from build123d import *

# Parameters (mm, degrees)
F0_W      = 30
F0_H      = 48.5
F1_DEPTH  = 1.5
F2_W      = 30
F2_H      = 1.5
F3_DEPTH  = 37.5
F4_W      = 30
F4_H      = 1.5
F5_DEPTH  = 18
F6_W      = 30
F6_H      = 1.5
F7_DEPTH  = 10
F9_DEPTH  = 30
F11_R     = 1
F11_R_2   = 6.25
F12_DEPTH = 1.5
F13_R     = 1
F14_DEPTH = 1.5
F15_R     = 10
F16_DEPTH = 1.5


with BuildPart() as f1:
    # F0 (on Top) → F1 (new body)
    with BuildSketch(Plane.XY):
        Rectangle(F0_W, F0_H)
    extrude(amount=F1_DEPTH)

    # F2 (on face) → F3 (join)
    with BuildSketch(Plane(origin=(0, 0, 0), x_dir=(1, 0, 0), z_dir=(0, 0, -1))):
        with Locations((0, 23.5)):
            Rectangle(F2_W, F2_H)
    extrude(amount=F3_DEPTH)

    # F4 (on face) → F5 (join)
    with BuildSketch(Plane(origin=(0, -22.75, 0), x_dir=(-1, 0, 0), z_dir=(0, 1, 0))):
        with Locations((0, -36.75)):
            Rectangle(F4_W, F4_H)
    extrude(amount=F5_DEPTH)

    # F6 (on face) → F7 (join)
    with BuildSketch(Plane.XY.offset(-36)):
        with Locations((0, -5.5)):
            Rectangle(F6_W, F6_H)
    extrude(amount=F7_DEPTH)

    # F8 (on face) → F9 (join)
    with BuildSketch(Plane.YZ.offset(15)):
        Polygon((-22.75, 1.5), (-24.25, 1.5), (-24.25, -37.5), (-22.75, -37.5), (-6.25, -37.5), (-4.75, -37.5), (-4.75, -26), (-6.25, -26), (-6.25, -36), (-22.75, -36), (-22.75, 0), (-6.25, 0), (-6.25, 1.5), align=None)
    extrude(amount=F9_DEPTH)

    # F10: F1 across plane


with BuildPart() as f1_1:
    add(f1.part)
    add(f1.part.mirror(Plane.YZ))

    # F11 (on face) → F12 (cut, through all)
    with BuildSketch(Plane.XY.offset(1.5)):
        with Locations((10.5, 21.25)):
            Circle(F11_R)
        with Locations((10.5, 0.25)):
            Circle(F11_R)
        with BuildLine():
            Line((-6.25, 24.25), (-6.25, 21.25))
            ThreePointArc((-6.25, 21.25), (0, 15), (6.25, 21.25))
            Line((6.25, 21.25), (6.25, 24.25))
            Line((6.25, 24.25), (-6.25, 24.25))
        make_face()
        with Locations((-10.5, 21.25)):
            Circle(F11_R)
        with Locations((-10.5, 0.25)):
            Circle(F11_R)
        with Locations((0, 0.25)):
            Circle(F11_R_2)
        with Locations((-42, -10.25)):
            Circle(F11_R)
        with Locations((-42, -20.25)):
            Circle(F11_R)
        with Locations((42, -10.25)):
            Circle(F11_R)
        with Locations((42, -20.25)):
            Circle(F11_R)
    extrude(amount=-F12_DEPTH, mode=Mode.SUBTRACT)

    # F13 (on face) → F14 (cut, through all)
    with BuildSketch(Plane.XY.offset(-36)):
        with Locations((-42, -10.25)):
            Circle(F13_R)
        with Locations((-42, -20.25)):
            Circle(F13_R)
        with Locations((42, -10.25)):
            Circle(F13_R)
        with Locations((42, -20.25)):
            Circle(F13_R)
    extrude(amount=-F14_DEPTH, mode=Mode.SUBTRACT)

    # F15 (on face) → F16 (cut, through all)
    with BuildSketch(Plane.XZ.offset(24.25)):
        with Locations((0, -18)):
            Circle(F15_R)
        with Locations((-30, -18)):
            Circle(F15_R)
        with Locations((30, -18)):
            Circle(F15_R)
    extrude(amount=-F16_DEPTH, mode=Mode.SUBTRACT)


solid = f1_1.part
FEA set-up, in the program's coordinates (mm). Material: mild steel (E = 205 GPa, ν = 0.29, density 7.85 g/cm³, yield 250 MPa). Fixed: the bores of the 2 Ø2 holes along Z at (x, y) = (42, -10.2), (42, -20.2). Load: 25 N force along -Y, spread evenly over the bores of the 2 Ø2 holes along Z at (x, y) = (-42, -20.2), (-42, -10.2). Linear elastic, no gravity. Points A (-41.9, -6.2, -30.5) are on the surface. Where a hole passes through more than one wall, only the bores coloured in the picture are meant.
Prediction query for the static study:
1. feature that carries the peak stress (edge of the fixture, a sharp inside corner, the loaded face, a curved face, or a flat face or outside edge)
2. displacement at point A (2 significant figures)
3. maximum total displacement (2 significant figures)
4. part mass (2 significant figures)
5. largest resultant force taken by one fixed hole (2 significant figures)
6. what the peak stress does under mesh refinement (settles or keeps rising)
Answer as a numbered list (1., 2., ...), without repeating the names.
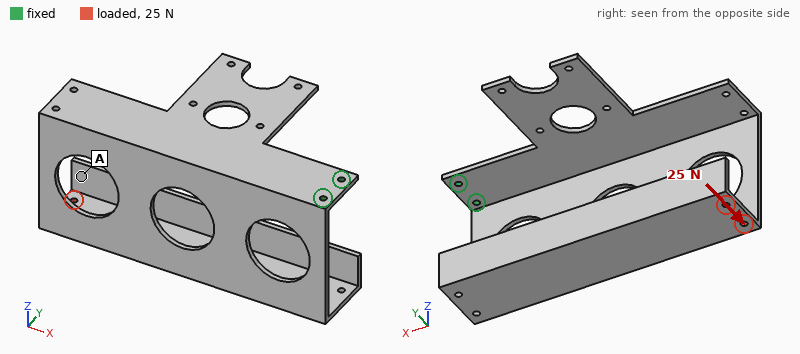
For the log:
1. edge of the fixture
2. 0.76 mm
3. 0.91 mm
4. 85 g
5. 200 N
6. keeps rising
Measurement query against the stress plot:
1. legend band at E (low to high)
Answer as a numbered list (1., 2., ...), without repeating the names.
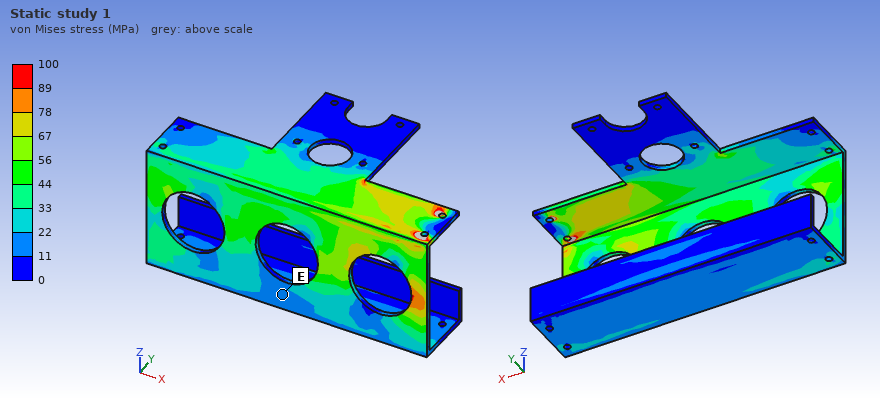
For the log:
1. 11 to 22 MPa
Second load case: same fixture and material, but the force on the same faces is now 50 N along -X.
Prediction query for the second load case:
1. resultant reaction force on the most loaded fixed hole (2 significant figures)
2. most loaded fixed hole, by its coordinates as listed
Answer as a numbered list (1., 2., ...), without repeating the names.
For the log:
1. 37 N
2. (42, -10.2)
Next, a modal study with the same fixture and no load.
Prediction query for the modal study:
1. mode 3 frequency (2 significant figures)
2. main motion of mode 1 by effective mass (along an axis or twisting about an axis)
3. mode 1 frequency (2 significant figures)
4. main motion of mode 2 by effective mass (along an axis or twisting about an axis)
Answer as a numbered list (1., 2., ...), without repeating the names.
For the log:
1. 490 Hz
2. along Y
3. 180 Hz
4. along Z
